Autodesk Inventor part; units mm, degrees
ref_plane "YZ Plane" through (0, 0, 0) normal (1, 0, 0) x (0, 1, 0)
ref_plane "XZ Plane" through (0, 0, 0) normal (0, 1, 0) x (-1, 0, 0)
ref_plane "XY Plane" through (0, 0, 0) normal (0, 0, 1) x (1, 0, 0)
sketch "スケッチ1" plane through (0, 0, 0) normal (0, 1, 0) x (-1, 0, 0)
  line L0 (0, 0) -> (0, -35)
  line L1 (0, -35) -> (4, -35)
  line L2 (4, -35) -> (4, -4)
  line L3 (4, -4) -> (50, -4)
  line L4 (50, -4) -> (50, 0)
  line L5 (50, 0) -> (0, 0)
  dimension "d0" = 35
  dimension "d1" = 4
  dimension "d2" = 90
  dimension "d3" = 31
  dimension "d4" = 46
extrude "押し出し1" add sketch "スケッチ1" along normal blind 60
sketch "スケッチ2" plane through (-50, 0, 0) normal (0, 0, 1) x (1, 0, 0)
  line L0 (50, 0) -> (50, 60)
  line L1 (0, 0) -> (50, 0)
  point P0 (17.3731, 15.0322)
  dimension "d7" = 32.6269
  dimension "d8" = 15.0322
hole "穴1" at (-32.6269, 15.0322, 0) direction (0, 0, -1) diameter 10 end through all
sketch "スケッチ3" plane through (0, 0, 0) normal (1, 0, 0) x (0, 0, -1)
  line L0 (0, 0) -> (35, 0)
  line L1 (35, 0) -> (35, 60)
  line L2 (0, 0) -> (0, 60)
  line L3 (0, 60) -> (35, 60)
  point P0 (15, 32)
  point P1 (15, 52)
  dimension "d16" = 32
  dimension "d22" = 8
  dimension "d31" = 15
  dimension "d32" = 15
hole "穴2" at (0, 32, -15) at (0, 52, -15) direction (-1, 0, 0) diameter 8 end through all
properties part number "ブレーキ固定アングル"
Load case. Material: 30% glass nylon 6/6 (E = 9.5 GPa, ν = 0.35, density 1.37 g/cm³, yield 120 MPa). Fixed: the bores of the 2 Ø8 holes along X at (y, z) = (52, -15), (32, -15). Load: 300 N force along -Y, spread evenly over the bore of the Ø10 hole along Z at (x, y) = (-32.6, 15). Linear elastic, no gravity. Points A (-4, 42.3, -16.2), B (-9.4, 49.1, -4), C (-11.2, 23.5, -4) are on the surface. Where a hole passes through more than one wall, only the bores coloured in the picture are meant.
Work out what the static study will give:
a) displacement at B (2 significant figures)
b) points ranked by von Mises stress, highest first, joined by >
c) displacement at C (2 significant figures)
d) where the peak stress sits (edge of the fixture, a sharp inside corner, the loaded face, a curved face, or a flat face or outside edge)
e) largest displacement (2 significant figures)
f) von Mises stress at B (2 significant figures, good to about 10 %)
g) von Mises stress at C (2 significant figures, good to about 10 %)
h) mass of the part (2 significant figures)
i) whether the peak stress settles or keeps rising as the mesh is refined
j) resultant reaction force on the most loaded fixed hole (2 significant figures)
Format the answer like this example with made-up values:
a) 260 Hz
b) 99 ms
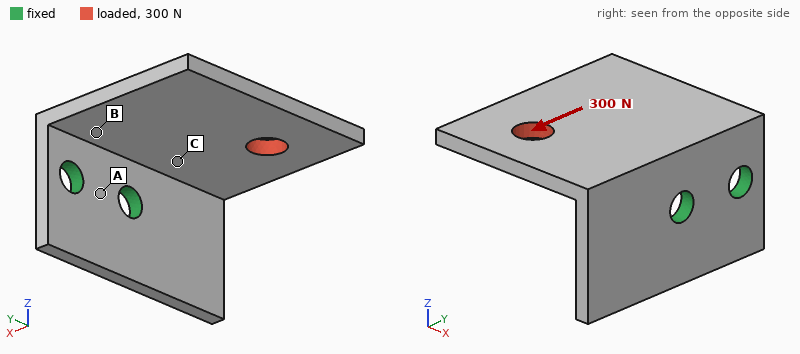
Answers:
a) 0.085 mm
b) B > C > A
c) 0.14 mm
d) edge of the fixture
e) 0.56 mm
f) 16 MPa
g) 8.9 MPa
h) 26 g
i) keeps rising
j) 400 N
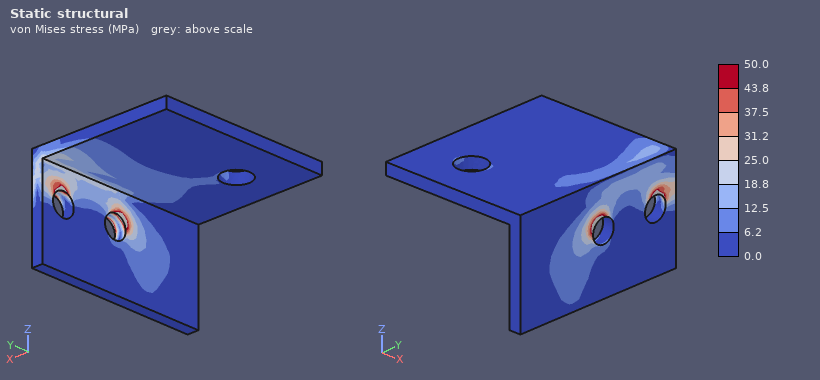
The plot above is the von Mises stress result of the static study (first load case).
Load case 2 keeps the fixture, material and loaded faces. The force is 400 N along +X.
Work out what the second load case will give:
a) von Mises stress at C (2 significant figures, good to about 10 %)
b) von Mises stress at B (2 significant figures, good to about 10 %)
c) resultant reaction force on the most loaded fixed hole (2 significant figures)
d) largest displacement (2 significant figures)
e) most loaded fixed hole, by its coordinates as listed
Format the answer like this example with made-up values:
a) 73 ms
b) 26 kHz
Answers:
a) 9.1 MPa
b) 14 MPa
c) 590 N
d) 0.94 mm
e) (32, -15)
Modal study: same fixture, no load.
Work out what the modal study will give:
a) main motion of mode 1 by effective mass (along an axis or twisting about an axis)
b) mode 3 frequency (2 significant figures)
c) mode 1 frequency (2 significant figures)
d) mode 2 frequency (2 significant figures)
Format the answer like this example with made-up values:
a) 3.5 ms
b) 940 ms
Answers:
a) along Z
b) 1500 Hz
c) 550 Hz
d) 1200 Hz
